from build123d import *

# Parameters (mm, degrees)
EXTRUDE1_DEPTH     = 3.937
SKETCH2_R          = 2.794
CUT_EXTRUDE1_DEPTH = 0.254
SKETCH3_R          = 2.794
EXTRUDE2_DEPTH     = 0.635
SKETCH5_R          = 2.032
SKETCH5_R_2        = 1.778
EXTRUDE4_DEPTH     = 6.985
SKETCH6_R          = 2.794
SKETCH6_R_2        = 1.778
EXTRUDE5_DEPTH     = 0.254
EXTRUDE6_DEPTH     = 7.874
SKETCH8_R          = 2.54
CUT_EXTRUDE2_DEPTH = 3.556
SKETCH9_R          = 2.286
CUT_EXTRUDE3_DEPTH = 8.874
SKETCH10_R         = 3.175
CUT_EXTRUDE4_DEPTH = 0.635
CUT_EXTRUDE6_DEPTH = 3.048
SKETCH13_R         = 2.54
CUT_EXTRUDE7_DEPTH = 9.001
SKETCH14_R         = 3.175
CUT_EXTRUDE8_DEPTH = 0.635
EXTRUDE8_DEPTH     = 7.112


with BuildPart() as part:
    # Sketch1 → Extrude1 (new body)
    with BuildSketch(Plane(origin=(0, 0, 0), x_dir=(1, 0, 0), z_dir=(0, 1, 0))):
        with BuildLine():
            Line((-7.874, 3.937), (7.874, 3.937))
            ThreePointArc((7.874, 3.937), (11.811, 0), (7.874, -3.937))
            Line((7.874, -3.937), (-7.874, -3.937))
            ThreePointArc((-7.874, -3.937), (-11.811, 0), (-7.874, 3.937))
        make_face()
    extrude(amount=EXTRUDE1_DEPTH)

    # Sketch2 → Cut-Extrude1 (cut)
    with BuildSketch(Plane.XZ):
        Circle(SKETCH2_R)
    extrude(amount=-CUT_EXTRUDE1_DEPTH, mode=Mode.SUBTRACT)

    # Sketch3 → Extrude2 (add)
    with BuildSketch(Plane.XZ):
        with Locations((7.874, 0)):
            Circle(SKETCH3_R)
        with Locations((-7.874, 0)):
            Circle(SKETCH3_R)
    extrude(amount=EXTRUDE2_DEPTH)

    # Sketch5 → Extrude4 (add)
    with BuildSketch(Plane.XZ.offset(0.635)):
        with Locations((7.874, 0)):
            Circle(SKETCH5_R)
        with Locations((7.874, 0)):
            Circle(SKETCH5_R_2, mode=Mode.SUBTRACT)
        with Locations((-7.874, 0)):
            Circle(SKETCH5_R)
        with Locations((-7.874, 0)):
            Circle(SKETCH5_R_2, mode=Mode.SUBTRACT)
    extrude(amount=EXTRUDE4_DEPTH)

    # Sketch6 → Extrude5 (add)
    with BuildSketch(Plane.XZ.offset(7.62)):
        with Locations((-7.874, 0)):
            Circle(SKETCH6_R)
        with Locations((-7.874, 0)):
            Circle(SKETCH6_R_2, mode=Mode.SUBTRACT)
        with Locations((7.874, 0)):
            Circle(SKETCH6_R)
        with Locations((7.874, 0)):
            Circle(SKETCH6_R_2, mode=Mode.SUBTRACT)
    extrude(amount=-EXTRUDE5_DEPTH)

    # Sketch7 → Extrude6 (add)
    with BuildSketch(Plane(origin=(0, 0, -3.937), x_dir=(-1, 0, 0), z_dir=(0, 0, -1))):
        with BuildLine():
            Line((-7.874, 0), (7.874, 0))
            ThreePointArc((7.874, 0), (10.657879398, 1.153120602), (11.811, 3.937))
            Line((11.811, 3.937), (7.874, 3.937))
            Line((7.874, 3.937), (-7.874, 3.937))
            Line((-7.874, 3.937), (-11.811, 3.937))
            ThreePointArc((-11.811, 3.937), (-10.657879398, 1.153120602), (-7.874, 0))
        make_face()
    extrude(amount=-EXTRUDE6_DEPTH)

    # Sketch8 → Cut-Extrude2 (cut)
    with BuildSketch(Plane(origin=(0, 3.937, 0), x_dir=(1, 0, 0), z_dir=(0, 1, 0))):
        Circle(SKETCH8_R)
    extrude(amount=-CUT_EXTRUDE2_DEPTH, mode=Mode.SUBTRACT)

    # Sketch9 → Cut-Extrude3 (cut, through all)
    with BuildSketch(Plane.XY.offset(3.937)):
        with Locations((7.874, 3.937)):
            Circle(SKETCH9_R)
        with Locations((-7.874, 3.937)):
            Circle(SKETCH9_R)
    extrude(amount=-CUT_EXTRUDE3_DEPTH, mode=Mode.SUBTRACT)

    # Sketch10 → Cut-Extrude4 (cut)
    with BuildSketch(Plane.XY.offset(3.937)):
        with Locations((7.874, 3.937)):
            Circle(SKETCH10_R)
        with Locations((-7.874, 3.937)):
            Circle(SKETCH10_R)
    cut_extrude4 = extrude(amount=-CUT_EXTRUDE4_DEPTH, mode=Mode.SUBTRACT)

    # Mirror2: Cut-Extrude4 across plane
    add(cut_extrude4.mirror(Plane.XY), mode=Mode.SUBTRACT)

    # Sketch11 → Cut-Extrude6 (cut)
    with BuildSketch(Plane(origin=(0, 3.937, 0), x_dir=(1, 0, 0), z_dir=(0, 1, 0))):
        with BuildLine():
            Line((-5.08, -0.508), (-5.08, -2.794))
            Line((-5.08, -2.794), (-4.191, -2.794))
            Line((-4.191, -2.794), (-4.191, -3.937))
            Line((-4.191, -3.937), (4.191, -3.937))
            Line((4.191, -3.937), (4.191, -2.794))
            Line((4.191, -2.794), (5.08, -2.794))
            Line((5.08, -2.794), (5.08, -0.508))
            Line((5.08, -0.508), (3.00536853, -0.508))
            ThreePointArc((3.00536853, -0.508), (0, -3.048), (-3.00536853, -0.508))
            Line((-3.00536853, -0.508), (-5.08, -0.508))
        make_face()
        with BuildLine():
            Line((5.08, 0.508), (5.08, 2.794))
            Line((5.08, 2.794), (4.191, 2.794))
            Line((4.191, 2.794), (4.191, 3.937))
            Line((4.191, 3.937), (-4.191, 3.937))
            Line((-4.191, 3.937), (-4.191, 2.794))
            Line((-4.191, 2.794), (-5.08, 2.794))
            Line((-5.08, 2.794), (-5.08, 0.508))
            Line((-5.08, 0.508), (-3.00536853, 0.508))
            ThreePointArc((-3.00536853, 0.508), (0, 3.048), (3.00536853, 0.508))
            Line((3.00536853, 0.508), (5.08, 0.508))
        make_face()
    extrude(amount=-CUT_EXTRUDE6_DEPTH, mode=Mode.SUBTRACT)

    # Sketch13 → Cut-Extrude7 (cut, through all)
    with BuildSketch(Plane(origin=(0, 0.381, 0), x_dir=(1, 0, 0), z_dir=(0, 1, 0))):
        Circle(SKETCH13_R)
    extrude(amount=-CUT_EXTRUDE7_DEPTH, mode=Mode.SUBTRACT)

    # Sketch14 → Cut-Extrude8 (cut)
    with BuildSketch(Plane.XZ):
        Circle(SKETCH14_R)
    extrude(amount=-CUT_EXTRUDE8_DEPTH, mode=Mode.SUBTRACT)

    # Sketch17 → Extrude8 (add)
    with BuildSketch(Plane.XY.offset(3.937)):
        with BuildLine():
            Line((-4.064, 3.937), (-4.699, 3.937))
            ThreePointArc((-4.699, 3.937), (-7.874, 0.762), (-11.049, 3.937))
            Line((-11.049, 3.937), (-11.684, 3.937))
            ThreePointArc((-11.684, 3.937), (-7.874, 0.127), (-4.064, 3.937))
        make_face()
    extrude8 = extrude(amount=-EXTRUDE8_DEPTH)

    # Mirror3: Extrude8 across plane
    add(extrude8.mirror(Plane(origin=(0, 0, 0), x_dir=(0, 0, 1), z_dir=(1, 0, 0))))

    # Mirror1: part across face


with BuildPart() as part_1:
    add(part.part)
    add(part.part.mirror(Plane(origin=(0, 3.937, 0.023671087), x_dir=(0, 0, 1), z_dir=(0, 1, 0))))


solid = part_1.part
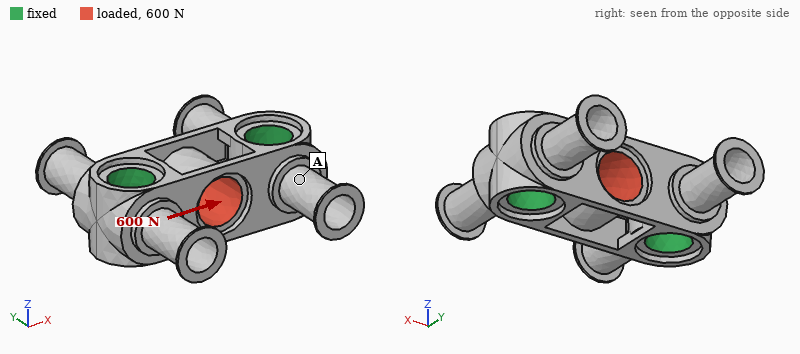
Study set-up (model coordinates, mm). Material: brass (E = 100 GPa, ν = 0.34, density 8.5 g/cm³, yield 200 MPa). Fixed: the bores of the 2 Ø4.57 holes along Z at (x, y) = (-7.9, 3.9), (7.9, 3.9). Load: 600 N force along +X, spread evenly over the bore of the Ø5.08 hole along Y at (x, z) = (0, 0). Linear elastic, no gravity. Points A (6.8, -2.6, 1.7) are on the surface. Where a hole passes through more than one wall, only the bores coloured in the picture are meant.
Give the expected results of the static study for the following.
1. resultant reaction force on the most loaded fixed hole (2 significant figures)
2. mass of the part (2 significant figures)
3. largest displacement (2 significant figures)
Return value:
300 N
7.4 g
4.3 µm
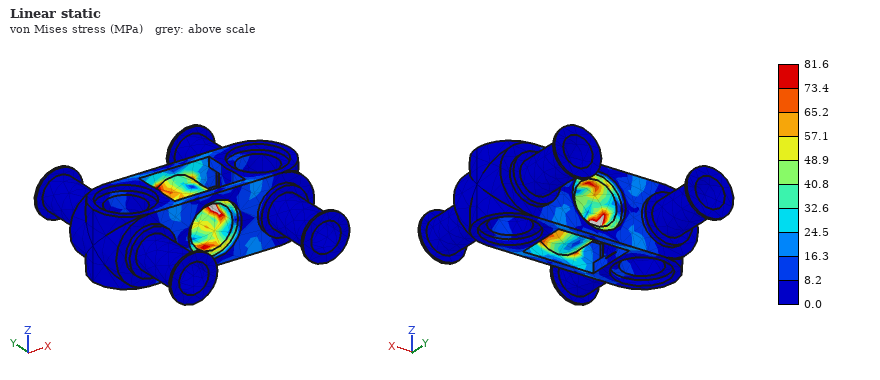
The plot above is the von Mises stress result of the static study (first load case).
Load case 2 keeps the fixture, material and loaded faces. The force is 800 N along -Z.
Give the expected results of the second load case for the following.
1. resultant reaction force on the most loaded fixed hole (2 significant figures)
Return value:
400 N
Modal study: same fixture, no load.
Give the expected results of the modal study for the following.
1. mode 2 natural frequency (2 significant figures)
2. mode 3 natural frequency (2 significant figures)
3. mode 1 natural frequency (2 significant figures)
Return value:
29 kHz
29 kHz
29 kHz
